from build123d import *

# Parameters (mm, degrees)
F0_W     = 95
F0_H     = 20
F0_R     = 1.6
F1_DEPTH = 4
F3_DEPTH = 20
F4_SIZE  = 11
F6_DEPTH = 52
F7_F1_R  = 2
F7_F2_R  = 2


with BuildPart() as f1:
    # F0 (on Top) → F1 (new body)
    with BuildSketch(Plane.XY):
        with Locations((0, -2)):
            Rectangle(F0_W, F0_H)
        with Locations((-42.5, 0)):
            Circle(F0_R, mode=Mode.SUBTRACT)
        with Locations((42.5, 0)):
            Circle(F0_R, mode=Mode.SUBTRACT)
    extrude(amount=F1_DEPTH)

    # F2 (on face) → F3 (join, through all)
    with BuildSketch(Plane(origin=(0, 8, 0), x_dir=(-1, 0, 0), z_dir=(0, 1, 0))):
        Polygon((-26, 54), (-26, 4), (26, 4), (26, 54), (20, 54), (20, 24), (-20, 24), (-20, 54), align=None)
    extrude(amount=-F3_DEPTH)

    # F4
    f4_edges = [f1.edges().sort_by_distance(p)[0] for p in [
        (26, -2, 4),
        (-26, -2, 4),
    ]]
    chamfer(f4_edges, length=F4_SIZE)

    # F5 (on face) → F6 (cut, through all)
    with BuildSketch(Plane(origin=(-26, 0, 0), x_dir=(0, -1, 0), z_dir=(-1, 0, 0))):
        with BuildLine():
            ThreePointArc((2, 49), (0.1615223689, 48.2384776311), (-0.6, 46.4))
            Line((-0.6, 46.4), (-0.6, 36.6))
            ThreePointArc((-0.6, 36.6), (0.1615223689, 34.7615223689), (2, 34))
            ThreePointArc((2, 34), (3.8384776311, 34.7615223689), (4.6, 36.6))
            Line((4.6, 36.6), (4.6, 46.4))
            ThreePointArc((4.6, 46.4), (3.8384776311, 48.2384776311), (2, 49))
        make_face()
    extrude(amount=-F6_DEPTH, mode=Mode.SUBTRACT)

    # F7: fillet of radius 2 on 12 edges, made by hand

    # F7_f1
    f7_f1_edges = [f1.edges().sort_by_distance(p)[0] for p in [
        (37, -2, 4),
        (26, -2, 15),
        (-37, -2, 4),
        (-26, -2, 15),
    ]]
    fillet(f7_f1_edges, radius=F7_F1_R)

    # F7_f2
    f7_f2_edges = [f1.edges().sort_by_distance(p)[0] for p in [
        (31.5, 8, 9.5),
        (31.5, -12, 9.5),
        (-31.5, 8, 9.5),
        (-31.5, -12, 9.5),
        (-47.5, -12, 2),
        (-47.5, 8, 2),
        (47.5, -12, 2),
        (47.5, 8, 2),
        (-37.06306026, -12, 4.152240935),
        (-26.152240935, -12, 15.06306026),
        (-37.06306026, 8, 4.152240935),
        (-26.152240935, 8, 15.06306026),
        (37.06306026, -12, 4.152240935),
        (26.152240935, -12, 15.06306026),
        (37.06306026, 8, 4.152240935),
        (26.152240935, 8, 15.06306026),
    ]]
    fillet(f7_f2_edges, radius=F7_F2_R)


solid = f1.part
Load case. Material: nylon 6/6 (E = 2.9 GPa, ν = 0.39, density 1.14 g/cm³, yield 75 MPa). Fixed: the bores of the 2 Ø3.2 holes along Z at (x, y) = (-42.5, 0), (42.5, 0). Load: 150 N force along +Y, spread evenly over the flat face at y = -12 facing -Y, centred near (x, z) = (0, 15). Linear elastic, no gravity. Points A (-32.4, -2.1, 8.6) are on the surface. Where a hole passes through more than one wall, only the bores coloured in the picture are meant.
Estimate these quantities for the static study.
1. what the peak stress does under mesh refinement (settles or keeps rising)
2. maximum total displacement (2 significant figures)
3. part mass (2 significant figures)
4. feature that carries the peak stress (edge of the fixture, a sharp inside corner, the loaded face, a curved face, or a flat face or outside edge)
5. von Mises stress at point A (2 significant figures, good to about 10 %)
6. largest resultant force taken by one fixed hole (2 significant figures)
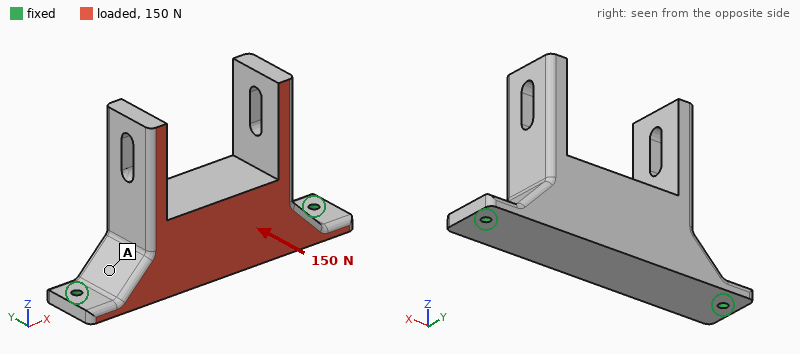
keeps rising
1.1 mm
42 g
edge of the fixture
4.4 MPa
80 N
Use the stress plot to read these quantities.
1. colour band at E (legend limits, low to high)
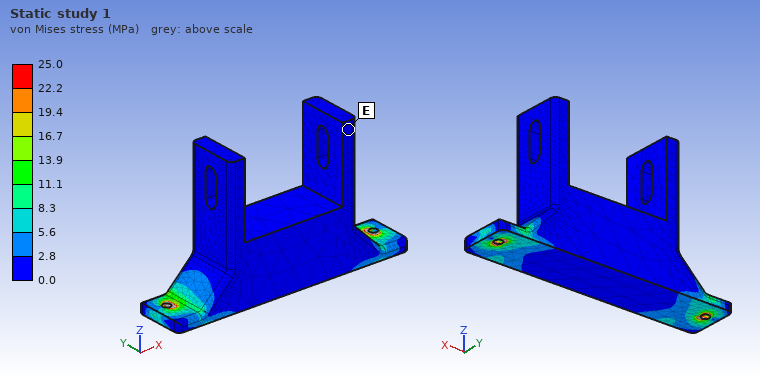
0.0 to 2.8 MPa
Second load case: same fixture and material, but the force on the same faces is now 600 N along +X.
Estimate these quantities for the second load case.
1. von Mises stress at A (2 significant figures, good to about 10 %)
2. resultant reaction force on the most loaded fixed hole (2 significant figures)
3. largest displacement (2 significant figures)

3.0 MPa
330 N
0.39 mm
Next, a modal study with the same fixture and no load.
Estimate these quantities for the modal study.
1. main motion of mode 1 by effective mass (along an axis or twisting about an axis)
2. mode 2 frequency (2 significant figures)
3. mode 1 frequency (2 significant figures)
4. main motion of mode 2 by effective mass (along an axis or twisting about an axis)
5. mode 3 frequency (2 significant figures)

along Y
1300 Hz
400 Hz
along X
1400 Hz
